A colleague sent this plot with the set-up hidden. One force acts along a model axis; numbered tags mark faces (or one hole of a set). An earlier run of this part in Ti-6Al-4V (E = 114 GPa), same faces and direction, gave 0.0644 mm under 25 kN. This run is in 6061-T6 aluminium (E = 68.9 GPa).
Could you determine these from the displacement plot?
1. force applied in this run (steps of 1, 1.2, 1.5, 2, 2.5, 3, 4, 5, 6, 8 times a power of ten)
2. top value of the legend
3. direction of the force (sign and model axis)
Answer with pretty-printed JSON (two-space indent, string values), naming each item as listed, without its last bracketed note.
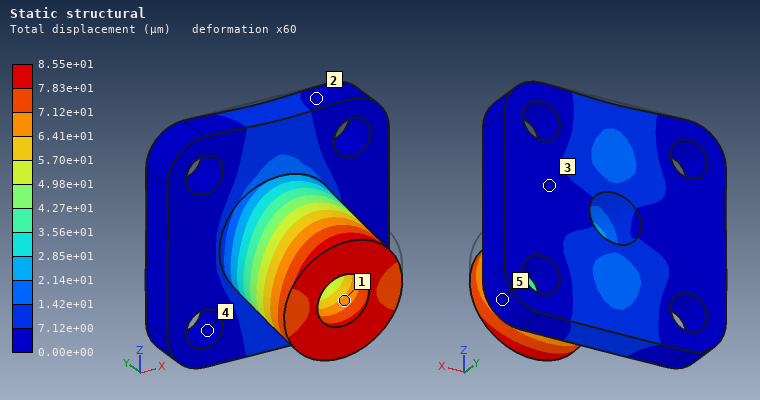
{
  "force applied in this run": "20 kN",
  "top value of the legend": "8.55e+01 µm",
  "direction of the force": "-Z"
}
